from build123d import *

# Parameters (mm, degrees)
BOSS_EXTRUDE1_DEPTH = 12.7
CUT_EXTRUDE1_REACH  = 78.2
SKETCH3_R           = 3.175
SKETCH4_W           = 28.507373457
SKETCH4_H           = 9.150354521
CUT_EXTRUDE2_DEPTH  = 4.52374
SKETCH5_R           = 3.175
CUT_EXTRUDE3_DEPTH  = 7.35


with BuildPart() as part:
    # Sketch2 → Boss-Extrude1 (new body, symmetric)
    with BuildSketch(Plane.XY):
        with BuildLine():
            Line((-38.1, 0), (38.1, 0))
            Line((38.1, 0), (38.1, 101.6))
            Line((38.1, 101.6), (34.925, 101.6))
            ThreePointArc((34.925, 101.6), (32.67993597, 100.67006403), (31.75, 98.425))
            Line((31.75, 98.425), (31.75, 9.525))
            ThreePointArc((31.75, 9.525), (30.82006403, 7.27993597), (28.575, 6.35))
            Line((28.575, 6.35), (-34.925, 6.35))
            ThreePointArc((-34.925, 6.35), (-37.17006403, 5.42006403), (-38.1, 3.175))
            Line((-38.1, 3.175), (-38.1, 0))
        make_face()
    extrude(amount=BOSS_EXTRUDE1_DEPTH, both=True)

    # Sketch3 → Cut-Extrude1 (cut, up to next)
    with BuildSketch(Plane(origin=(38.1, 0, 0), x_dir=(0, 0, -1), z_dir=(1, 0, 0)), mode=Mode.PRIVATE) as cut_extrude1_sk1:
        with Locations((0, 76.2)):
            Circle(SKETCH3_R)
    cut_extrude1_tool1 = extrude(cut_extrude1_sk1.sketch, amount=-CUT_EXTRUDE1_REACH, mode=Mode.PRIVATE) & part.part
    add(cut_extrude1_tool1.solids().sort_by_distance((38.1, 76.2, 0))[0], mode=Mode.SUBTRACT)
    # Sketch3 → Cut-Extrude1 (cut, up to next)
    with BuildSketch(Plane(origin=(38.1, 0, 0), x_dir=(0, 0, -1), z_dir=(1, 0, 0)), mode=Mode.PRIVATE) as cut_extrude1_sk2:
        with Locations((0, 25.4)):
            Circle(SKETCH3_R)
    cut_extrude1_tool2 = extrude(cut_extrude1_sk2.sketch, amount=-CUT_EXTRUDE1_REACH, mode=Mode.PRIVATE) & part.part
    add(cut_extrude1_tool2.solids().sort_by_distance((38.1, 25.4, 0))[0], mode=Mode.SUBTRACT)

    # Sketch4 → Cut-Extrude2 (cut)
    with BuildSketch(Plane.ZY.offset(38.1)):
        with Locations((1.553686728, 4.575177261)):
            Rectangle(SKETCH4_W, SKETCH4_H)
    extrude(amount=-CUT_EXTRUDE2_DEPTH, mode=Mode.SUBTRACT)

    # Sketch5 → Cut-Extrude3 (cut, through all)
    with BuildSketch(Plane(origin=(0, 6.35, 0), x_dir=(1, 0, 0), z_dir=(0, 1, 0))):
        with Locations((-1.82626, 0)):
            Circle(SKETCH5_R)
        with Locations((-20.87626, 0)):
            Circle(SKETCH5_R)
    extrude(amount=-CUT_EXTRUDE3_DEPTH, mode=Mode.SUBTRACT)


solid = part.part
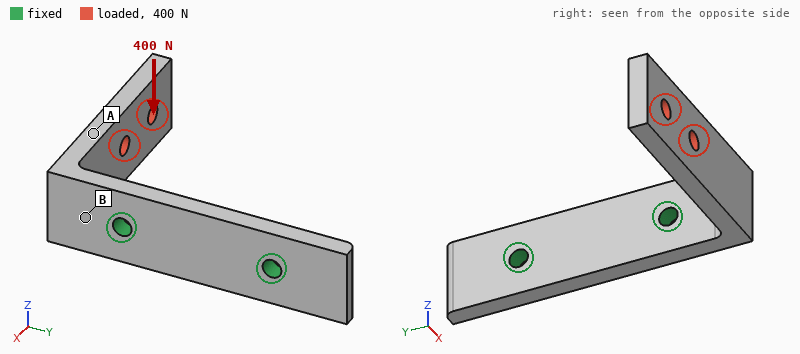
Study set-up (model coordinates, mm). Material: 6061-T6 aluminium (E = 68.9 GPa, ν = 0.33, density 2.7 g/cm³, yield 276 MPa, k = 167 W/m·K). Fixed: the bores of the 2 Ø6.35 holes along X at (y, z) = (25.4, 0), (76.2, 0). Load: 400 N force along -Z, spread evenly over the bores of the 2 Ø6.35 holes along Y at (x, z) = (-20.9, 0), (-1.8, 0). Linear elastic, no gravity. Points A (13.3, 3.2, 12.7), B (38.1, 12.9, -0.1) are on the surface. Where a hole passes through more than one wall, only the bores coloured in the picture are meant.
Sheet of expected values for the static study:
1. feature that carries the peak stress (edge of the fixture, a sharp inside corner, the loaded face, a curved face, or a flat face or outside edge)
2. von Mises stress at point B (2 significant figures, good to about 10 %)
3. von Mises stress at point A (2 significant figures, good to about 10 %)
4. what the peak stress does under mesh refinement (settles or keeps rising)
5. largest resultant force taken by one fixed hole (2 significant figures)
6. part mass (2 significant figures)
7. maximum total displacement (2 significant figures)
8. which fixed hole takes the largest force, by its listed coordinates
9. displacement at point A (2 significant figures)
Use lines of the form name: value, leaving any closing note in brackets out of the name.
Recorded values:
feature that carries the peak stress: edge of the fixture
von Mises stress at point B: 74 MPa
von Mises stress at point A: 15 MPa
what the peak stress does under mesh refinement: keeps rising
largest resultant force taken by one fixed hole: 510 N
part mass: 71 g
maximum total displacement: 0.47 mm
which fixed hole takes the largest force, by its listed coordinates: (25.4, 0)
displacement at point A: 0.17 mm
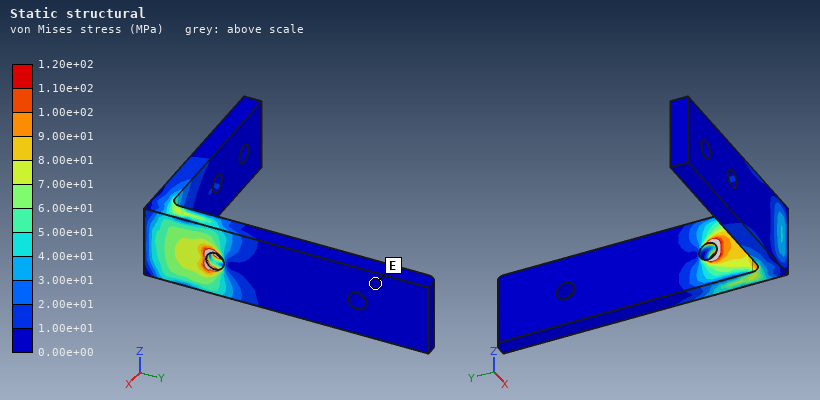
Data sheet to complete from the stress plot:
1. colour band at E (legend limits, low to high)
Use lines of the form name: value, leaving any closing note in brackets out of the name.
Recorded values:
colour band at E: 0.00e+00 to 1.00e+01 MPa
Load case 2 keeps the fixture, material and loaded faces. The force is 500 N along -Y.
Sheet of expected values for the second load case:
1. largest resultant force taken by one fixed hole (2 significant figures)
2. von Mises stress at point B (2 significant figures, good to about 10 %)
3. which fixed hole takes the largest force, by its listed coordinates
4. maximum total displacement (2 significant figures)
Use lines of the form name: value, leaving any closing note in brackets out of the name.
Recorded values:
largest resultant force taken by one fixed hole: 470 N
von Mises stress at point B: 120 MPa
which fixed hole takes the largest force, by its listed coordinates: (25.4, 0)
maximum total displacement: 1.5 mm
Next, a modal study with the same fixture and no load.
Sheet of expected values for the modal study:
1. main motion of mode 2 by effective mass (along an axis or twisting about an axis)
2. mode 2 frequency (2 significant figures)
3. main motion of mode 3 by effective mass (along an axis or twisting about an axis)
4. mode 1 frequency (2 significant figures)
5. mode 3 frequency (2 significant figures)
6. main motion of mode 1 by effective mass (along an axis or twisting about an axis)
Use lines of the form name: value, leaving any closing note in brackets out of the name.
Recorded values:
main motion of mode 2 by effective mass: along Z
mode 2 frequency: 1200 Hz
main motion of mode 3 by effective mass: along X
mode 1 frequency: 790 Hz
mode 3 frequency: 3600 Hz
main motion of mode 1 by effective mass: along Y
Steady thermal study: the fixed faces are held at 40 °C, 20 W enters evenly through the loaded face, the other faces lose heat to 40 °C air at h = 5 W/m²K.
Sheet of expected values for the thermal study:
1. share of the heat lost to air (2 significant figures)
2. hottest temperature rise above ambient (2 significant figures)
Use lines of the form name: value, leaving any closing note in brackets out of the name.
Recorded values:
share of the heat lost to air: 4.2 %
hottest temperature rise above ambient: 50 K
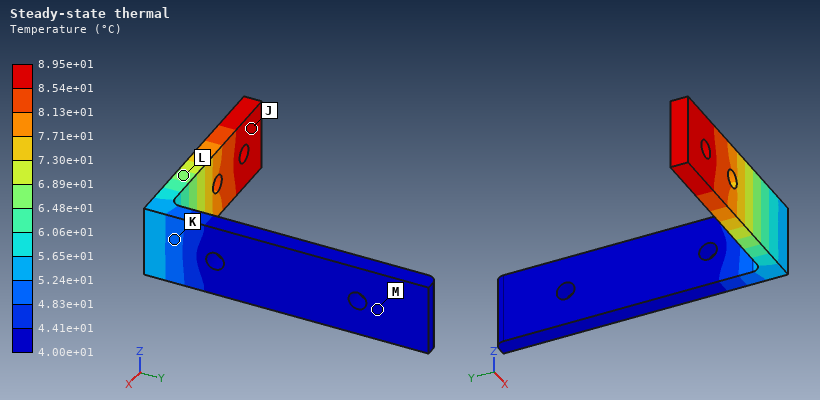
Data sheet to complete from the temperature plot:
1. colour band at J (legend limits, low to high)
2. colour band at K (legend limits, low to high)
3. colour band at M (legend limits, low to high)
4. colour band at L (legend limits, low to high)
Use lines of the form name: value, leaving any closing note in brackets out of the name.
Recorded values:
colour band at J: 8.54e+01 to 8.95e+01 °C
colour band at K: 4.83e+01 to 5.24e+01 °C
colour band at M: 4.00e+01 to 4.41e+01 °C
colour band at L: 6.48e+01 to 6.89e+01 °C
